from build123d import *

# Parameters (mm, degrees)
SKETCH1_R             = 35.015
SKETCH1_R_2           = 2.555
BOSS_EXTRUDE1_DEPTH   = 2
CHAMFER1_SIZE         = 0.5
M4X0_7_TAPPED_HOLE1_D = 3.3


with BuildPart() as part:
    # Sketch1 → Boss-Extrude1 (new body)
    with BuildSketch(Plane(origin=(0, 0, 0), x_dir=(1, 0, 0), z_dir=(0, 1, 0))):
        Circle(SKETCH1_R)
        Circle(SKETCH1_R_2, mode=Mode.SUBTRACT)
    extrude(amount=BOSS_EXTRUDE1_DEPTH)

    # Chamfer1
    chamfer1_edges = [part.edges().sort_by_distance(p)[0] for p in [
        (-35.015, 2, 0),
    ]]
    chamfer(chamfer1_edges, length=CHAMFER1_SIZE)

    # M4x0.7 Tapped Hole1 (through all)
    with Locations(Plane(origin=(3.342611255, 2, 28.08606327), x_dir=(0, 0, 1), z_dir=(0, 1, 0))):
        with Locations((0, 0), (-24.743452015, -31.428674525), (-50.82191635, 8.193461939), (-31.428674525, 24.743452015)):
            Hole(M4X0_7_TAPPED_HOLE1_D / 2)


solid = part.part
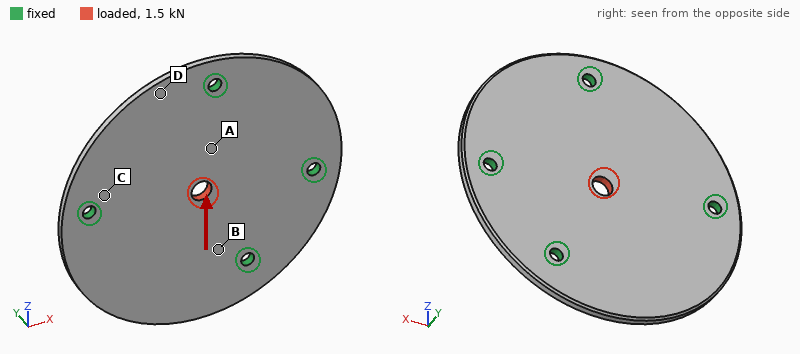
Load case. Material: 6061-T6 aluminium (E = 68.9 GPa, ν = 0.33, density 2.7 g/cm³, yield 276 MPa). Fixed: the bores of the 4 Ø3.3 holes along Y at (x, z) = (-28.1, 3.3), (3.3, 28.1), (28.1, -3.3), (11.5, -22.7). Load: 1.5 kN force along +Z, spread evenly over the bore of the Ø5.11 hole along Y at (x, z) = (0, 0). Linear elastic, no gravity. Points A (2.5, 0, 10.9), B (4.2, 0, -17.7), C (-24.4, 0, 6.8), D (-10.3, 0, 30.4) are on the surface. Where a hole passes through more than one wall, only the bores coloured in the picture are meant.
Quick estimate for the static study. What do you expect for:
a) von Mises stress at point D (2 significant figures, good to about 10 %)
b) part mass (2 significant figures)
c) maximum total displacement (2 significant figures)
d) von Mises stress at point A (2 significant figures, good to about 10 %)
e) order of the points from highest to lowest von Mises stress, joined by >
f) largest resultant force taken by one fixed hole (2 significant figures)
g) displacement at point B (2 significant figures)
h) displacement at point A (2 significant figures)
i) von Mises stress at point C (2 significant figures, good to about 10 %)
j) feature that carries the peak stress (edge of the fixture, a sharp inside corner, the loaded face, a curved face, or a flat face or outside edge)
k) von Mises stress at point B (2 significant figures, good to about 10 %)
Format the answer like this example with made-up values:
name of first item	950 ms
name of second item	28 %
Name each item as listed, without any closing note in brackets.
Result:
von Mises stress at point D	5.0 MPa
part mass	20 g
maximum total displacement	9.7 µm
von Mises stress at point A	23 MPa
order of the points from highest to lowest von Mises stress, joined by >	A > B > C > D
largest resultant force taken by one fixed hole	490 N
displacement at point B	3.4 µm
displacement at point A	5.0 µm
von Mises stress at point C	9.7 MPa
feature that carries the peak stress	the loaded face
von Mises stress at point B	16 MPa
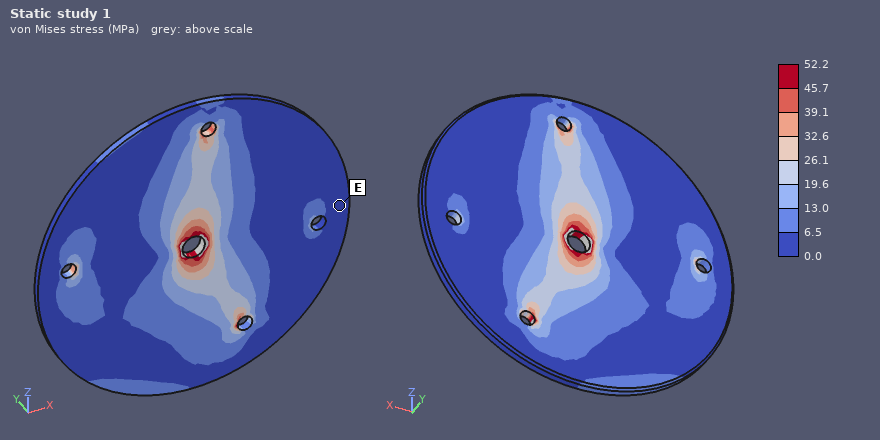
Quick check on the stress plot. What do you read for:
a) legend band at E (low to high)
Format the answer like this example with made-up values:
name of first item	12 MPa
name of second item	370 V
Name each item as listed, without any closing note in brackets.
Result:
legend band at E	0.0 to 6.5 MPa
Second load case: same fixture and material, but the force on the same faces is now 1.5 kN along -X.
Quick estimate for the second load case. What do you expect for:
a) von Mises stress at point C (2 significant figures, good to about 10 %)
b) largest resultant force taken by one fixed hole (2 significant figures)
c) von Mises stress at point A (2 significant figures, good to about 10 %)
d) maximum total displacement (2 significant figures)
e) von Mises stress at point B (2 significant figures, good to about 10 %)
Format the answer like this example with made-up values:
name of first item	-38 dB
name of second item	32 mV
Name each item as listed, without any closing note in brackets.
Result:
von Mises stress at point C	14 MPa
largest resultant force taken by one fixed hole	460 N
von Mises stress at point A	6.0 MPa
maximum total displacement	9.0 µm
von Mises stress at point B	8.0 MPa
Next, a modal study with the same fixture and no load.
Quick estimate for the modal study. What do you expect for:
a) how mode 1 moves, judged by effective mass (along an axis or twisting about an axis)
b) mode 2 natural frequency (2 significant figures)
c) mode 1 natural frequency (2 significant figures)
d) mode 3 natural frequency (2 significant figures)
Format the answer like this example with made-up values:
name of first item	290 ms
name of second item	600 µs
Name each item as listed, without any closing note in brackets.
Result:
how mode 1 moves, judged by effective mass	along Y
mode 2 natural frequency	5000 Hz
mode 1 natural frequency	2900 Hz
mode 3 natural frequency	5100 Hz
